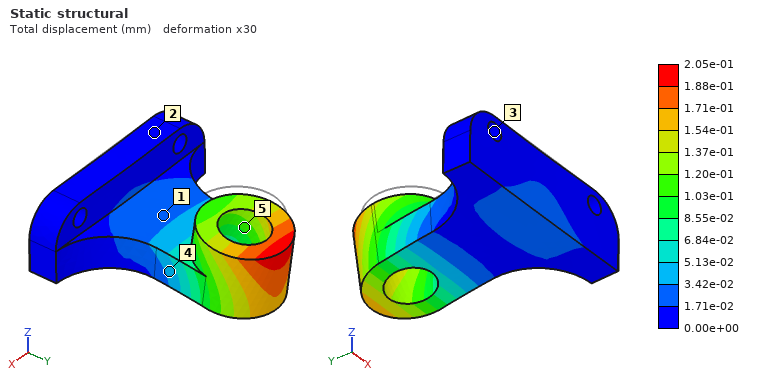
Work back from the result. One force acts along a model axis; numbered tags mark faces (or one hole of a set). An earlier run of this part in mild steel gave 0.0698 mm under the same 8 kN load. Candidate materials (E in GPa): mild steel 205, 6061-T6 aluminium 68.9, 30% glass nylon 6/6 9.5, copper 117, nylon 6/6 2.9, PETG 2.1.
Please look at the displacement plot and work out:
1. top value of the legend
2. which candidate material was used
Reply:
2.05e-01 mm
6061-T6 aluminium
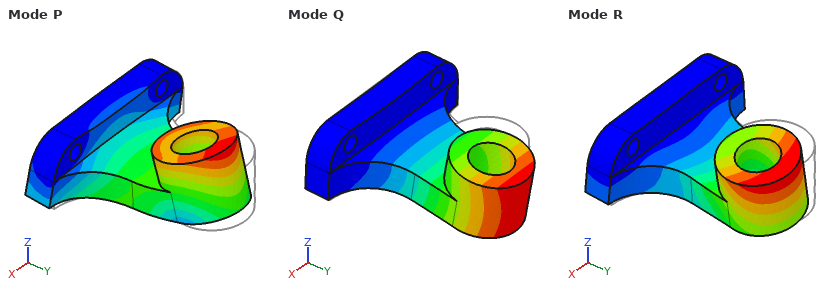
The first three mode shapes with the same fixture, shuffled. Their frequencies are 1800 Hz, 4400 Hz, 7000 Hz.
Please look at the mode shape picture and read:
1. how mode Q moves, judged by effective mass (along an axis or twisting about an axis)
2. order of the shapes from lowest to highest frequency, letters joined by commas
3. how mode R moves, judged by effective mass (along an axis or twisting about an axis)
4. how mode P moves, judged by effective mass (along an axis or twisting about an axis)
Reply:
along Z
Q, R, P
along X
along Y
